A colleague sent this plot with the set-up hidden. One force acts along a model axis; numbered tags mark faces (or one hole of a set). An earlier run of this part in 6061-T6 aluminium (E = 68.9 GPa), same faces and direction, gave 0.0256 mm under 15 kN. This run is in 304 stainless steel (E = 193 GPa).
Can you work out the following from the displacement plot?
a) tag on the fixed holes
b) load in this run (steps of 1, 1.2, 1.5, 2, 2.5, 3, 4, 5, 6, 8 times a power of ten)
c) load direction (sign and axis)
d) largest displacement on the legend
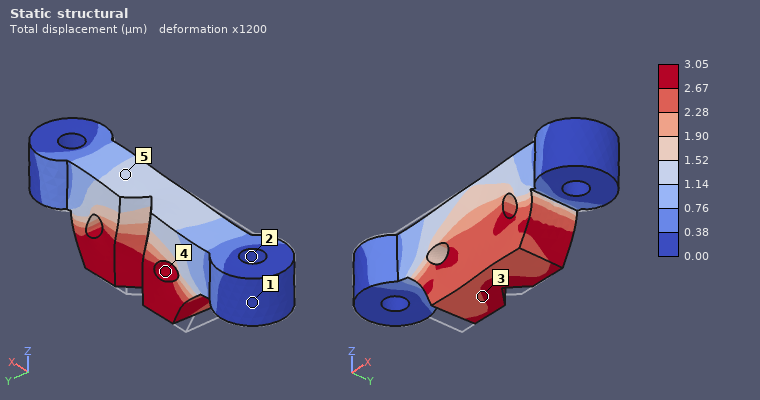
2
5 kN
+X
3.05 µm
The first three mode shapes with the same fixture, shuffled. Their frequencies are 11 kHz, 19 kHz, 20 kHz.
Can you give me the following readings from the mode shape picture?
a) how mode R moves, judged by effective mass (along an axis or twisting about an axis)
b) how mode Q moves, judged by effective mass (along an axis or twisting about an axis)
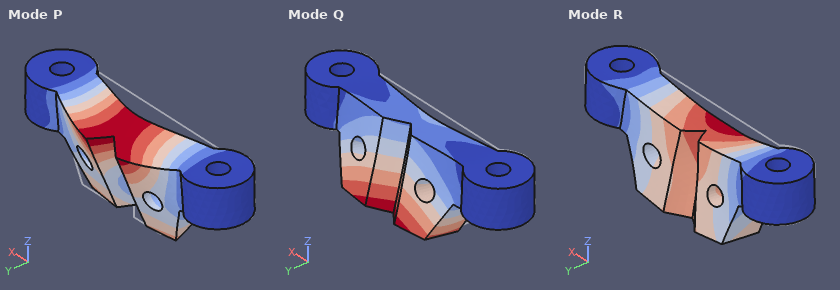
along Z
along Y
